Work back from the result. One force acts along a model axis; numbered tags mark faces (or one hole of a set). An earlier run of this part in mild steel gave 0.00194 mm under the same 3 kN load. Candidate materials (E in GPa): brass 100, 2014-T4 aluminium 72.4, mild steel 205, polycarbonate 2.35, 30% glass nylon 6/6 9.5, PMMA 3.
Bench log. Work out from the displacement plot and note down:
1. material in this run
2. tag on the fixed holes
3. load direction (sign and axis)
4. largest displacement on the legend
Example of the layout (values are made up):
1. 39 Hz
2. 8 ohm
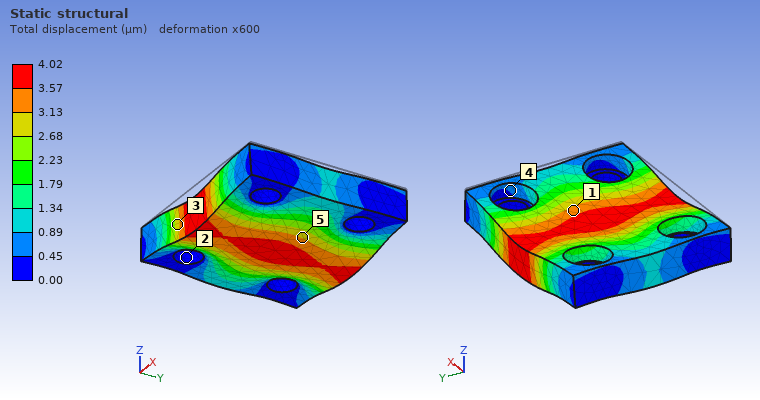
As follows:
1. brass
2. 2
3. -Z
4. 4.02 µm
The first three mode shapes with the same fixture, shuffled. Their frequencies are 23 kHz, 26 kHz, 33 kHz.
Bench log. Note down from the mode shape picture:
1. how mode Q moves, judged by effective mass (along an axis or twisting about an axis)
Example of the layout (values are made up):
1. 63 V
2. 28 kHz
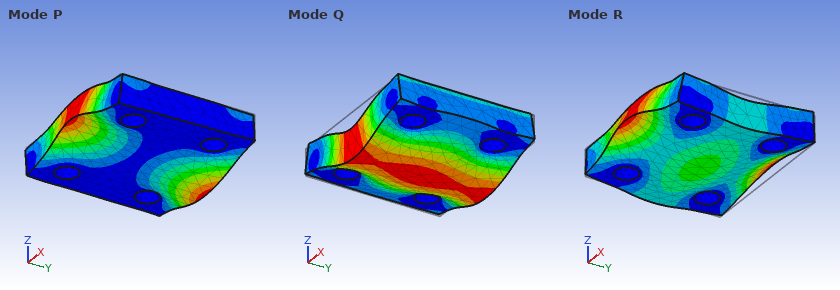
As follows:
1. along Z
